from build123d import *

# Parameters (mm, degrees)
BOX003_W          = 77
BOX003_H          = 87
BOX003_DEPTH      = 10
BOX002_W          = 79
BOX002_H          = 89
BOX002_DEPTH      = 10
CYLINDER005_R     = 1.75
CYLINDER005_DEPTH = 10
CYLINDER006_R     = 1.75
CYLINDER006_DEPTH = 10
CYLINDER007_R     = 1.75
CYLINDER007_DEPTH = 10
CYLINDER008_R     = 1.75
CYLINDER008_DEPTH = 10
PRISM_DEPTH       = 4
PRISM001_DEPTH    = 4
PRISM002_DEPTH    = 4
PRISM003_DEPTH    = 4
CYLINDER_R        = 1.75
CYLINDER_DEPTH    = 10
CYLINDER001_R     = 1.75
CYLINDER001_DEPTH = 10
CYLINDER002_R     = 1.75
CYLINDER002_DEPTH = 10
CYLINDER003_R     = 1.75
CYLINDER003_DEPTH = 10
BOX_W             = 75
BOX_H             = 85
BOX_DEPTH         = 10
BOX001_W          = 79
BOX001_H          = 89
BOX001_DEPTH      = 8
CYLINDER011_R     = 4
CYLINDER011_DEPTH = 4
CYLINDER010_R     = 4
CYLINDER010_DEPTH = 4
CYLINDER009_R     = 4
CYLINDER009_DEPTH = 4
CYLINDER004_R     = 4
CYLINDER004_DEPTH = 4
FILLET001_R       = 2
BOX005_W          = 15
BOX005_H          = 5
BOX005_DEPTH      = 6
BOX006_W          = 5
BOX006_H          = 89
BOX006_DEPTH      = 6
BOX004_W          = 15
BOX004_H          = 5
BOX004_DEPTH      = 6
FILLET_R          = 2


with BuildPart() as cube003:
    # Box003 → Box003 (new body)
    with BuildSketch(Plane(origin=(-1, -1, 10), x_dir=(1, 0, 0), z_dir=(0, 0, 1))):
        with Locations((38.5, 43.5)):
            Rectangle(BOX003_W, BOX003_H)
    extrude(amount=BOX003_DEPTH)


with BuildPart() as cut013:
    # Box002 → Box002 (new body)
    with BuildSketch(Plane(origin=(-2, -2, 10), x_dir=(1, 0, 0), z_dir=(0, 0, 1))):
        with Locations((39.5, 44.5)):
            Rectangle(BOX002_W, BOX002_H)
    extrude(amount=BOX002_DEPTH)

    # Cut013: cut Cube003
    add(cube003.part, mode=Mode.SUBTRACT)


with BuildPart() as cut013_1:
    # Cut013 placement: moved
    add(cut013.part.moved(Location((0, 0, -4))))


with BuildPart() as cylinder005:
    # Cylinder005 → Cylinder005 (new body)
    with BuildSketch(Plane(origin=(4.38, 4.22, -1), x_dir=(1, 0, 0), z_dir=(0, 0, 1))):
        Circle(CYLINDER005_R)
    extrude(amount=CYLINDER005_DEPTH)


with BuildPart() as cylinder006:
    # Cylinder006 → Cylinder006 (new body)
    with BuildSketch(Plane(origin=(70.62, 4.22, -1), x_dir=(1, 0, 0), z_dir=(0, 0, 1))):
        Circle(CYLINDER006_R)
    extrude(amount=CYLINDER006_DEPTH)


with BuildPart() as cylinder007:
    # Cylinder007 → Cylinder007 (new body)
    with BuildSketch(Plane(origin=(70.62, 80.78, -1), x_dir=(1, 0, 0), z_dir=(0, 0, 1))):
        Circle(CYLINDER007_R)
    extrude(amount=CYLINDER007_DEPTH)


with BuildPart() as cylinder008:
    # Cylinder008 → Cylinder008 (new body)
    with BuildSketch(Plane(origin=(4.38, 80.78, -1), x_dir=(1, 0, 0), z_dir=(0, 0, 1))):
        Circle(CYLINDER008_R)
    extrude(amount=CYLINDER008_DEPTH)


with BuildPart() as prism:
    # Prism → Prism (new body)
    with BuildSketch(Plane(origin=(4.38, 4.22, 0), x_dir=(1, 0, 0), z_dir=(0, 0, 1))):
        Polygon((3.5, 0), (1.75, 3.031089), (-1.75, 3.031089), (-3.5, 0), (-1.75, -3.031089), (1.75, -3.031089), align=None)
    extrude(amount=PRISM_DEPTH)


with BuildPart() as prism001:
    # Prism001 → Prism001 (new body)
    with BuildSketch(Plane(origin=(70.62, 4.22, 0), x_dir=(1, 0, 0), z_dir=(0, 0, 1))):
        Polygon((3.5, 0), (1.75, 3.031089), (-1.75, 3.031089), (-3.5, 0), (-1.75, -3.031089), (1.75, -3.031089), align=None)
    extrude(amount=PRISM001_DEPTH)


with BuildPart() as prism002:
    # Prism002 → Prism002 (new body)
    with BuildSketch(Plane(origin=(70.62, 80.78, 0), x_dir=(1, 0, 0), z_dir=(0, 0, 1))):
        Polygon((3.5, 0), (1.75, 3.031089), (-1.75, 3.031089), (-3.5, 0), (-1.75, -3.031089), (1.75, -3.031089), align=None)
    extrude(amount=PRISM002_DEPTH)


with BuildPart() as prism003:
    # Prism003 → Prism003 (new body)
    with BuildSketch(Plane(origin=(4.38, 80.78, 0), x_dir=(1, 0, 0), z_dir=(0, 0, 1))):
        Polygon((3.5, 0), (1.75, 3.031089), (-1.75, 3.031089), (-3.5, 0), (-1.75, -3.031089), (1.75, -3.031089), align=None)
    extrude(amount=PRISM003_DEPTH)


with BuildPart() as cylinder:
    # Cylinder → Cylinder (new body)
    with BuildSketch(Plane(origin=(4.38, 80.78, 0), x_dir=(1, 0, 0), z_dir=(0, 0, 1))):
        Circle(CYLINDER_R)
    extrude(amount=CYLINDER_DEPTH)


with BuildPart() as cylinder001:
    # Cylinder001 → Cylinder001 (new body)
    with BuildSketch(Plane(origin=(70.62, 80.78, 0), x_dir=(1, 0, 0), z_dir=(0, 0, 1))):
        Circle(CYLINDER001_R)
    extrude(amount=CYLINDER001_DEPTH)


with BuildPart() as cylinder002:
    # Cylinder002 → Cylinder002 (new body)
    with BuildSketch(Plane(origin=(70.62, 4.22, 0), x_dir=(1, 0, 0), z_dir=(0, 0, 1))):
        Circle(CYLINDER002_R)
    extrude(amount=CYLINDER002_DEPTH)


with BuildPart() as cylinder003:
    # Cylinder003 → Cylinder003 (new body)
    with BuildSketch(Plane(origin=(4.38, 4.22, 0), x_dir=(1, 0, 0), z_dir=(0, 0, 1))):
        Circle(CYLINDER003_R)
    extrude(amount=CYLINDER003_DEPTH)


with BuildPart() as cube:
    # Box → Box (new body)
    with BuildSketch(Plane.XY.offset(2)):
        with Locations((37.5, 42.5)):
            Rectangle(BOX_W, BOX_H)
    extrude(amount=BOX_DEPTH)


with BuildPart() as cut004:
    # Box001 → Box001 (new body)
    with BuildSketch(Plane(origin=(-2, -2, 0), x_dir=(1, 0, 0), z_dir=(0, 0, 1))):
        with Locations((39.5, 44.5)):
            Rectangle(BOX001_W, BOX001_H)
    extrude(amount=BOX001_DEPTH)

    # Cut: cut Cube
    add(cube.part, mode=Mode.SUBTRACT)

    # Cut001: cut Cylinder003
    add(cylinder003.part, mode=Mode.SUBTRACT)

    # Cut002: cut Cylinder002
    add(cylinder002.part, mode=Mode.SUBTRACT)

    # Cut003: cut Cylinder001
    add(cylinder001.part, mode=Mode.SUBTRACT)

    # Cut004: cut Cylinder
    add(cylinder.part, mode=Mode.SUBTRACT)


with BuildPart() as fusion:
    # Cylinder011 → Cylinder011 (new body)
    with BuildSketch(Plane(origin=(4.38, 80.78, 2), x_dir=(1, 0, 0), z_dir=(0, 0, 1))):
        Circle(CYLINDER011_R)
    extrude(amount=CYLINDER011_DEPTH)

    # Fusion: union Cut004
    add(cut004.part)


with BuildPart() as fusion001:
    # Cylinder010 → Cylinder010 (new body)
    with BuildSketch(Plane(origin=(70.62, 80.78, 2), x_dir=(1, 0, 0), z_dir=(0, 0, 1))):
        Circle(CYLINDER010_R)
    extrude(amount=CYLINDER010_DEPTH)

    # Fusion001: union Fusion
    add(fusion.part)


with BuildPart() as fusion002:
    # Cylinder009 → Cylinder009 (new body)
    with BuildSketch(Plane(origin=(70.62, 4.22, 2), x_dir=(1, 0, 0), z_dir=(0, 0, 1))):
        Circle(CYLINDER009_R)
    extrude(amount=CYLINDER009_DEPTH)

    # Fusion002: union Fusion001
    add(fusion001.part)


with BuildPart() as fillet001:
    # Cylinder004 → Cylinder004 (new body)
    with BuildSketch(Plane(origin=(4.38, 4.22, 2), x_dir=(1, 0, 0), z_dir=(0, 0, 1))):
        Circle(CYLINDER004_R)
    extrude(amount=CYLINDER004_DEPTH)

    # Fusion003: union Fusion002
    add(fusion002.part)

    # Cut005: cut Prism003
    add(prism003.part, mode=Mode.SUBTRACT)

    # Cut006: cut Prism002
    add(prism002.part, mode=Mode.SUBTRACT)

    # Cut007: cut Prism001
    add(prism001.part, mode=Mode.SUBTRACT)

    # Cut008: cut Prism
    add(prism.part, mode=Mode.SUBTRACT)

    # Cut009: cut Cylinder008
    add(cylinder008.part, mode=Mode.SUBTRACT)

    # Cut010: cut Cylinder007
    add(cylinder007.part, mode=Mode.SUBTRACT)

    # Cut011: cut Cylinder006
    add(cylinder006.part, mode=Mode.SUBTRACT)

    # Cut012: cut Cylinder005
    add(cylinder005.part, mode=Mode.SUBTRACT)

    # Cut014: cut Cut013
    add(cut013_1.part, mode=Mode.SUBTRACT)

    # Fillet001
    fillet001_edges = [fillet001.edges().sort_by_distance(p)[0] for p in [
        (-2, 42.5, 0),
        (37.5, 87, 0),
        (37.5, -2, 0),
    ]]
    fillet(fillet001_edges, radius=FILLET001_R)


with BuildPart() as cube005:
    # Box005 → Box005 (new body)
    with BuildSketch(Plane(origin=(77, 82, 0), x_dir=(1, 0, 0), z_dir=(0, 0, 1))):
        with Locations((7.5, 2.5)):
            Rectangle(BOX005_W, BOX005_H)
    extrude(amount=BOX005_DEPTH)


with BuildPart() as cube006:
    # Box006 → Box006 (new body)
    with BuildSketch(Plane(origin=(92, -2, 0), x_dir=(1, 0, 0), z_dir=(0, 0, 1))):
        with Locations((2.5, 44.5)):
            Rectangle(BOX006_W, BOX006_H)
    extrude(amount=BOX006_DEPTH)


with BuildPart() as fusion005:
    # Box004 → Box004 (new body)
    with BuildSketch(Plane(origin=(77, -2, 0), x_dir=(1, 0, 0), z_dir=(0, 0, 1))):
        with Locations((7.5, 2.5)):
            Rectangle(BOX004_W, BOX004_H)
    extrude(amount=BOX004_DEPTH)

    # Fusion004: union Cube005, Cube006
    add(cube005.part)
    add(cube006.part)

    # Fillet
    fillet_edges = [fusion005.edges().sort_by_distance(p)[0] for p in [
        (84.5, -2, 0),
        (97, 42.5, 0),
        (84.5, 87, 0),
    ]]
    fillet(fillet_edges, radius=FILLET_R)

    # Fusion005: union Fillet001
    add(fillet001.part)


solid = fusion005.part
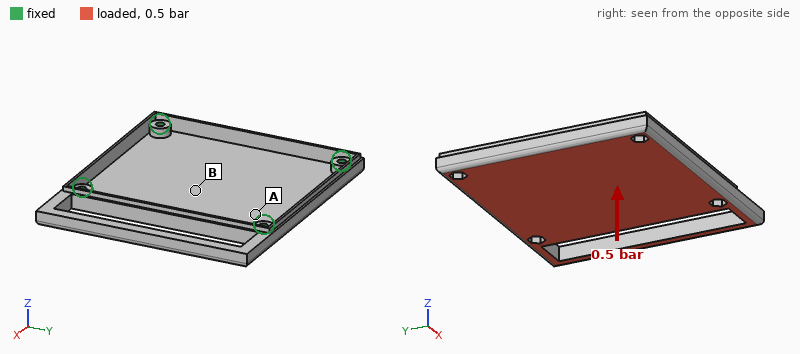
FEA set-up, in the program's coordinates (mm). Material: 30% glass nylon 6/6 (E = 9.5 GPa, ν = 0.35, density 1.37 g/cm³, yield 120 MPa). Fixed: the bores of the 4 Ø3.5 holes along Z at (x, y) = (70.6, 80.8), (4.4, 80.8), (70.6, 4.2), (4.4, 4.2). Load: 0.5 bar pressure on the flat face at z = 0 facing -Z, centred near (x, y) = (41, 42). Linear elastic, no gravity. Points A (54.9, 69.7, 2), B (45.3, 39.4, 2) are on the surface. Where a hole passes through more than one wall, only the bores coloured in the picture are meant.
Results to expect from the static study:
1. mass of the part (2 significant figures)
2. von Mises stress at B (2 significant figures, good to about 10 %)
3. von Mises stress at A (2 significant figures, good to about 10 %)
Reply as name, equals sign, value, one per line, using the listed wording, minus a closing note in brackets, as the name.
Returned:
mass of the part = 28 g
von Mises stress at B = 17 MPa
von Mises stress at A = 7.4 MPa
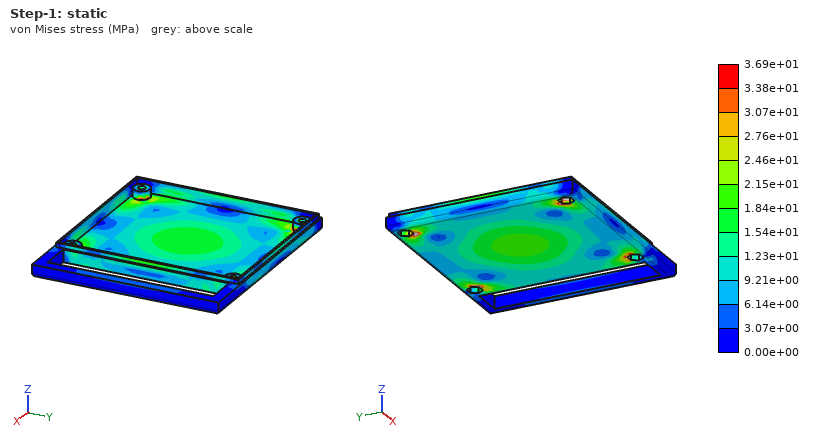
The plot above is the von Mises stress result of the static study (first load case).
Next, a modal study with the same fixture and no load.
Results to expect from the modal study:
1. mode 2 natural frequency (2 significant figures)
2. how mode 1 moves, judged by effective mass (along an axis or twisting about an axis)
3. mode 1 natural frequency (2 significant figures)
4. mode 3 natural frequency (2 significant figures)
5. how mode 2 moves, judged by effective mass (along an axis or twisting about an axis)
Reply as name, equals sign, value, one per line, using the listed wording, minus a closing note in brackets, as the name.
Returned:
mode 2 natural frequency = 900 Hz
how mode 1 moves, judged by effective mass = along Z
mode 1 natural frequency = 860 Hz
mode 3 natural frequency = 1600 Hz
how mode 2 moves, judged by effective mass = along Z
